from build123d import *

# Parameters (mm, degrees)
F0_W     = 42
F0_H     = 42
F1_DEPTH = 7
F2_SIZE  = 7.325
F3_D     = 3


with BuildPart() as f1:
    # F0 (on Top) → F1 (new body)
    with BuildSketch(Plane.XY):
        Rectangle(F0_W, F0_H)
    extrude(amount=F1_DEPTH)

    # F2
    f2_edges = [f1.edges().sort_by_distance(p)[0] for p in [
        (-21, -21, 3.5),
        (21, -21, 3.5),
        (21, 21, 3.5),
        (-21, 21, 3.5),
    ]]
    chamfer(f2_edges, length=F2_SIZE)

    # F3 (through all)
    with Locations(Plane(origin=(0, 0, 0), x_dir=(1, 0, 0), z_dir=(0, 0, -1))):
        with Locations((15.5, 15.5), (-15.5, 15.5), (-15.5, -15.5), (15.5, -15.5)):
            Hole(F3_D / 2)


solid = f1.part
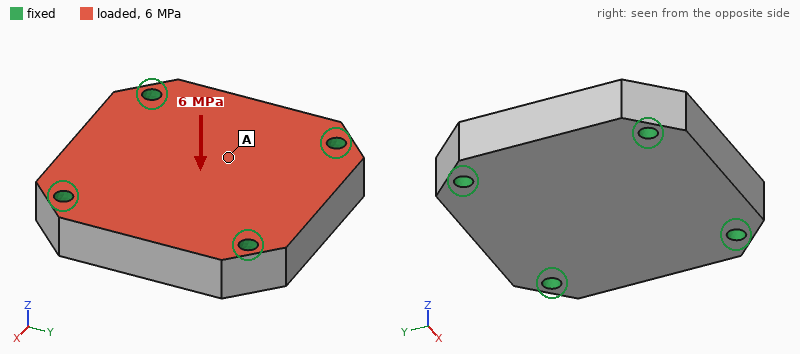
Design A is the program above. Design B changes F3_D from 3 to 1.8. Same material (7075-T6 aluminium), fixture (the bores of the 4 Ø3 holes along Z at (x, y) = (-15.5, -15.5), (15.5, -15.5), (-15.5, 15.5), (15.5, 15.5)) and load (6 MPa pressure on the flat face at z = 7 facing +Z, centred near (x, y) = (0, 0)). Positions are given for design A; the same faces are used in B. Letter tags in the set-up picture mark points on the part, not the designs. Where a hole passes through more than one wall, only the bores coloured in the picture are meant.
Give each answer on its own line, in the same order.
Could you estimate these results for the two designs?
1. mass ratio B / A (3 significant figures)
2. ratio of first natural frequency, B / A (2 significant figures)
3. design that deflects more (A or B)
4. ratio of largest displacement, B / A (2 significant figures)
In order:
1.01
0.90
B
1.2
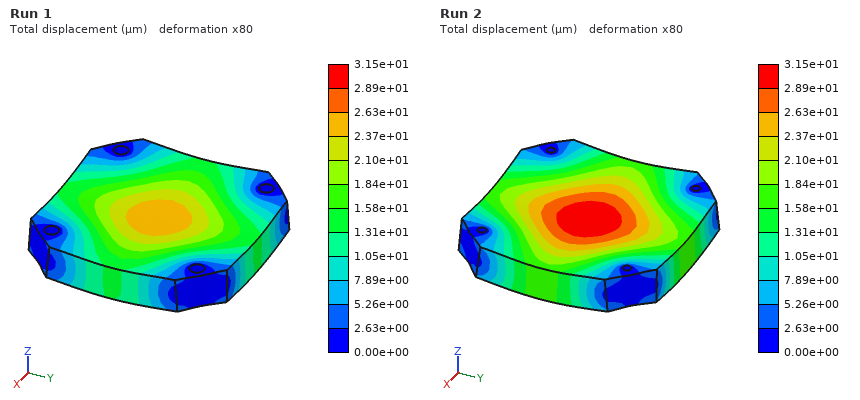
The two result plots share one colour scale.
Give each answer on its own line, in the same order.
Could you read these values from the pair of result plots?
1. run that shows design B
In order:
Run 2
